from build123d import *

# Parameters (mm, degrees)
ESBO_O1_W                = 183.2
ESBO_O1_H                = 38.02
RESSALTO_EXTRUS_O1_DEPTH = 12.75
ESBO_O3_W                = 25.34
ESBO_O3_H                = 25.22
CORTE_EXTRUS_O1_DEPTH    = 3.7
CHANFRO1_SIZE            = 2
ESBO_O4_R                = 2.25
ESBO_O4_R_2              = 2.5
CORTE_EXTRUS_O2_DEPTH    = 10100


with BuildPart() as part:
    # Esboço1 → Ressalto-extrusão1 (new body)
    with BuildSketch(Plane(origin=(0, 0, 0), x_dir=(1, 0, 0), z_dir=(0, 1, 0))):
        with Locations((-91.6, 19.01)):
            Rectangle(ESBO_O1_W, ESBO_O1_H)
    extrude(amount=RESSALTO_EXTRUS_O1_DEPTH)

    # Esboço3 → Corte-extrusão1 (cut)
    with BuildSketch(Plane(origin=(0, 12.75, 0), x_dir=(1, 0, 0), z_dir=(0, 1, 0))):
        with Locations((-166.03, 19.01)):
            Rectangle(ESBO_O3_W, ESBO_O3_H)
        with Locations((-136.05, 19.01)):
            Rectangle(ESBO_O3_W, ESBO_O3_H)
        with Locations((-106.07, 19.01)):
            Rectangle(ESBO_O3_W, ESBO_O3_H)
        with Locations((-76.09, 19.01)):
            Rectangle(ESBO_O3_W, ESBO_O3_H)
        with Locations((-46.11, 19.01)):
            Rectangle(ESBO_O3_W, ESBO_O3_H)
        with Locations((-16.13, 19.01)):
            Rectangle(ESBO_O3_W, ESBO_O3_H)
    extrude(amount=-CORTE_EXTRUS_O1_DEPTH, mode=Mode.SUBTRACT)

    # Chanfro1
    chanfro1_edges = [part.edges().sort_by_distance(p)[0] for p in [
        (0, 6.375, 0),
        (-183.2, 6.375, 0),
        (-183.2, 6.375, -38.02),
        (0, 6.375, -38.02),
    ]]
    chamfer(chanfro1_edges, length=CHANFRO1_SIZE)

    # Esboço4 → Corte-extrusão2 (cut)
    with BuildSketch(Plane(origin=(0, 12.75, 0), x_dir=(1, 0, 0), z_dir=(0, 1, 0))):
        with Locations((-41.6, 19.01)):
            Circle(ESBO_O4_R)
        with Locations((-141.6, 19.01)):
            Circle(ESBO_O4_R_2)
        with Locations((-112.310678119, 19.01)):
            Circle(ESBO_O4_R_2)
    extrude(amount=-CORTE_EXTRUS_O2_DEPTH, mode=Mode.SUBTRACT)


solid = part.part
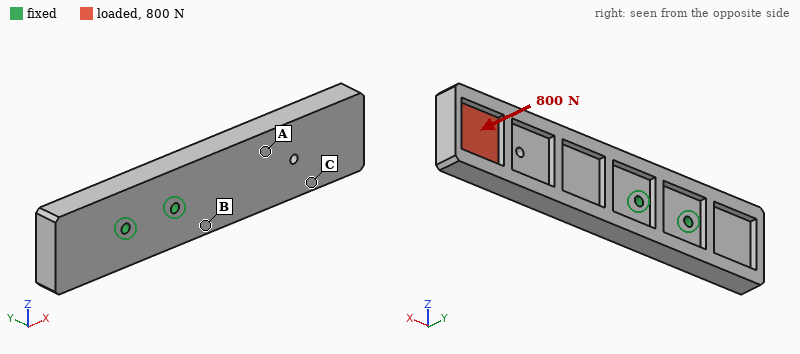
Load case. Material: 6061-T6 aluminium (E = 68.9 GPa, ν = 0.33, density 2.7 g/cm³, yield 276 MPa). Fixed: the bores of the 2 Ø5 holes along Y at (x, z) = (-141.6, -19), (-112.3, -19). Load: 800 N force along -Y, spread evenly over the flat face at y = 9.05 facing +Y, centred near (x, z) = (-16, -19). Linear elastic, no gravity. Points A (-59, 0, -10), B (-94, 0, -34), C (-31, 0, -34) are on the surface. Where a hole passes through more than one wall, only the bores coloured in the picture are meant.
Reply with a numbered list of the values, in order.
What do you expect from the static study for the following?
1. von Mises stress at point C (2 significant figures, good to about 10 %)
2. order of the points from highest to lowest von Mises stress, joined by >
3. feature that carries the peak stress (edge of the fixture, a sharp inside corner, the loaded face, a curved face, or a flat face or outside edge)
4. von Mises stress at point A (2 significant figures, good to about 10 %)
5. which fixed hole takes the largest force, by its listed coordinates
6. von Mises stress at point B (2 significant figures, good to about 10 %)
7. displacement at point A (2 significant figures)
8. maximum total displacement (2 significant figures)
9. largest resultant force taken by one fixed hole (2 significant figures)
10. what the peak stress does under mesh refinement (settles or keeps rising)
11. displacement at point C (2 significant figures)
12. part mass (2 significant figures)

1. 16 MPa
2. B > A > C
3. edge of the fixture
4. 43 MPa
5. (-112.3, -19)
6. 78 MPa
7. 0.39 mm
8. 1.2 mm
9. 2.4 kN
10. keeps rising
11. 0.75 mm
12. 200 g
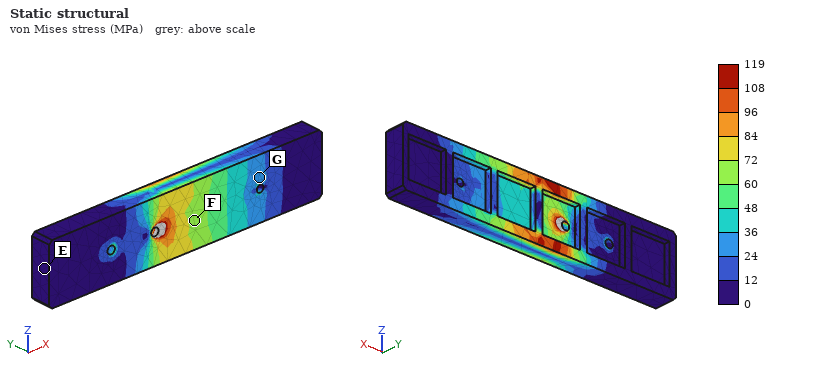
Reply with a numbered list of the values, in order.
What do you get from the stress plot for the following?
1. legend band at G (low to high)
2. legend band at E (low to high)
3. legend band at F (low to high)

1. 24 to 36 MPa
2. 0 to 12 MPa
3. 60 to 72 MPa
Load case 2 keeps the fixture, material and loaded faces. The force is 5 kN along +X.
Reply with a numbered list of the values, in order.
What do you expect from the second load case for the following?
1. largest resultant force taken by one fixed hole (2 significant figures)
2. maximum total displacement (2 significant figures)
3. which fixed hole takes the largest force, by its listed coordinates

1. 3.5 kN
2. 0.46 mm
3. (-112.3, -19)
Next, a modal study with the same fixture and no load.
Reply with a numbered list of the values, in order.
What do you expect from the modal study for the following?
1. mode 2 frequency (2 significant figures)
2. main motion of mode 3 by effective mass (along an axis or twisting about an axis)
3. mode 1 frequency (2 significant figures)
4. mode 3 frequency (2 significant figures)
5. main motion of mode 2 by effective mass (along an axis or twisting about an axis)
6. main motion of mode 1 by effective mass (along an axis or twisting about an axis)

1. 1700 Hz
2. twisting about X
3. 660 Hz
4. 2800 Hz
5. along Z
6. along Y
